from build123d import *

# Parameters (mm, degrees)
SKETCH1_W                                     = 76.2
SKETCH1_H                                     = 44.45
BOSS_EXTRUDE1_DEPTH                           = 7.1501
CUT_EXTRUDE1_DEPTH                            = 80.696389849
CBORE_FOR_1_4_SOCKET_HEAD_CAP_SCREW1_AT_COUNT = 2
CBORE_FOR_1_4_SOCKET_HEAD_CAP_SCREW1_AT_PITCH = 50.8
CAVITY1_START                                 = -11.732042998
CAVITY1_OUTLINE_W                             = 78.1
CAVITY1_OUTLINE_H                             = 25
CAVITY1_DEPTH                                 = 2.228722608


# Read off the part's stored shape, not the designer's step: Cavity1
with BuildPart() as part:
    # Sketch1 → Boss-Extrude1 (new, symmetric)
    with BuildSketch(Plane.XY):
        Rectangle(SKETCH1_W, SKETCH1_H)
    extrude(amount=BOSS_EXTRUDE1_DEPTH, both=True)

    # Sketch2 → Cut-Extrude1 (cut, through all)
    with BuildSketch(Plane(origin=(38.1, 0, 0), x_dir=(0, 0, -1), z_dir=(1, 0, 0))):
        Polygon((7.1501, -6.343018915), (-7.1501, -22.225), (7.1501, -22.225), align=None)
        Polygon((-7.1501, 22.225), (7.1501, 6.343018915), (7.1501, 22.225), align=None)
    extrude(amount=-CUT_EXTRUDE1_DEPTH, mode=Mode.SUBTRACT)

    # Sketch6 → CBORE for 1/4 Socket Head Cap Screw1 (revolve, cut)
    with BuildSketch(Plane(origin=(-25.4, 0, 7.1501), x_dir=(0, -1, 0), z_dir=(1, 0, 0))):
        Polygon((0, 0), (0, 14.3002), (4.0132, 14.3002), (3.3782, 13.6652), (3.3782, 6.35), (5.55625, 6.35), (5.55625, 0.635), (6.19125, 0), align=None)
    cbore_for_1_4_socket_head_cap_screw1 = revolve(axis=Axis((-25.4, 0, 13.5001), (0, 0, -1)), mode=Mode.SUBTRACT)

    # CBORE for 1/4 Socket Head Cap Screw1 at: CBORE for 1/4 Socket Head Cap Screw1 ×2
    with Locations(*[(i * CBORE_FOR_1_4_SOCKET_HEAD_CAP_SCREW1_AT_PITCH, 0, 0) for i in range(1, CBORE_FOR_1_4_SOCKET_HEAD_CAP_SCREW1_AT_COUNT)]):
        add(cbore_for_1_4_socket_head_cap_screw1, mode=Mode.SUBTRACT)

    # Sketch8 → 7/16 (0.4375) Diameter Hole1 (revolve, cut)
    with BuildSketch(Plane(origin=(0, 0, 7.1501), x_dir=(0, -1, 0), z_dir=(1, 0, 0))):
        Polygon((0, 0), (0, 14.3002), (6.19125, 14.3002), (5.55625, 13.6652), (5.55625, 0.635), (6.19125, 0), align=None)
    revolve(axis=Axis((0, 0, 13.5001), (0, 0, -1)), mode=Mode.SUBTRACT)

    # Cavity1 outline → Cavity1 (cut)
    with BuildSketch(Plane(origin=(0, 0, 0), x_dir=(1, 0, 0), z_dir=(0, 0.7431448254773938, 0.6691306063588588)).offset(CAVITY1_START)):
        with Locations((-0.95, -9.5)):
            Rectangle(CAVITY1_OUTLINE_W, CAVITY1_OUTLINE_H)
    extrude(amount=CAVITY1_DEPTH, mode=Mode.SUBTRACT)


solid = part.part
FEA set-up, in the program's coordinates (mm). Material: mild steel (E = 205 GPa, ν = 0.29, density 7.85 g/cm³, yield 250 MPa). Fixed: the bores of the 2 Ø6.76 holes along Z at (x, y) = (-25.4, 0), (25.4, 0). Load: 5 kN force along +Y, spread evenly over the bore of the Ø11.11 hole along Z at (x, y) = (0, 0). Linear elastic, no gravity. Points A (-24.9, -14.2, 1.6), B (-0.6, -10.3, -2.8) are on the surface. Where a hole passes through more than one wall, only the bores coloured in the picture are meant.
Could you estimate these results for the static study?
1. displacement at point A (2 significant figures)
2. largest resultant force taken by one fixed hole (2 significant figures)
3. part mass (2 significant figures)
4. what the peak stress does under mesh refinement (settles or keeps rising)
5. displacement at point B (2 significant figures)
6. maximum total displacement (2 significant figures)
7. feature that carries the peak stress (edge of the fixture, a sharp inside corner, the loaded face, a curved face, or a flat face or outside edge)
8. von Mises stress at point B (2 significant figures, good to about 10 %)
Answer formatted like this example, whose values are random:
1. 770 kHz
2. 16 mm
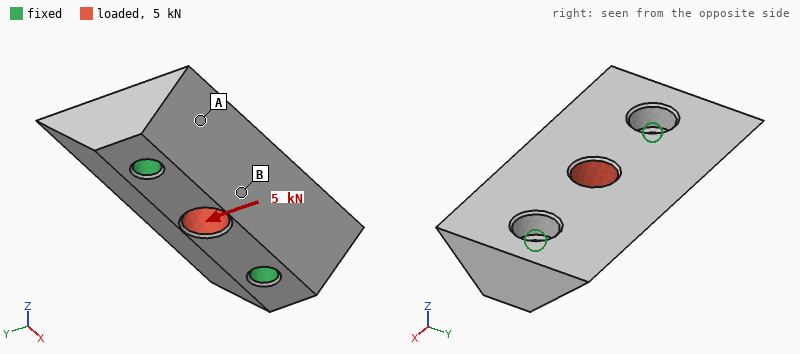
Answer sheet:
1. 2.3 µm
2. 2.5 kN
3. 210 g
4. keeps rising
5. 4.3 µm
6. 5.9 µm
7. edge of the fixture
8. 31 MPa
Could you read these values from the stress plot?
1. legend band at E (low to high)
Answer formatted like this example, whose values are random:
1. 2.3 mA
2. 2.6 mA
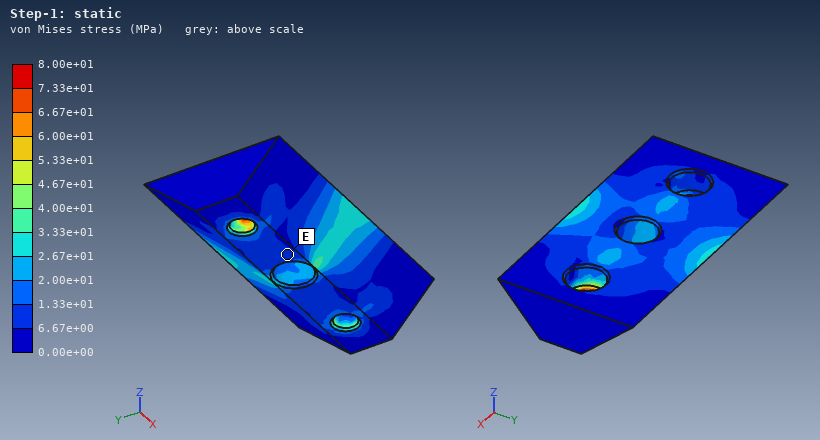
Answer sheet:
1. 6.67e+00 to 1.33e+01 MPa
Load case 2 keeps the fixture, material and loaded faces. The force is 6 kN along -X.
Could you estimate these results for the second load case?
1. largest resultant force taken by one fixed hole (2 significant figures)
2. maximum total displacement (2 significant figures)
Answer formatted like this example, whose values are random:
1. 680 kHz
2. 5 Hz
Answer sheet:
1. 3.0 kN
2. 1.9 µm
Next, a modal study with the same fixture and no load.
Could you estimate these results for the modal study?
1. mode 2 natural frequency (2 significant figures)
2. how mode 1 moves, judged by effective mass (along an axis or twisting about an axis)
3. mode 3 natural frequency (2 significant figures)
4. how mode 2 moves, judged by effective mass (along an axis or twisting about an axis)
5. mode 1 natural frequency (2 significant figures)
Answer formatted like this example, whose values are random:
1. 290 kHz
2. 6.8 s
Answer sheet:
1. 15 kHz
2. along Y
3. 17 kHz
4. along Z
5. 11 kHz
